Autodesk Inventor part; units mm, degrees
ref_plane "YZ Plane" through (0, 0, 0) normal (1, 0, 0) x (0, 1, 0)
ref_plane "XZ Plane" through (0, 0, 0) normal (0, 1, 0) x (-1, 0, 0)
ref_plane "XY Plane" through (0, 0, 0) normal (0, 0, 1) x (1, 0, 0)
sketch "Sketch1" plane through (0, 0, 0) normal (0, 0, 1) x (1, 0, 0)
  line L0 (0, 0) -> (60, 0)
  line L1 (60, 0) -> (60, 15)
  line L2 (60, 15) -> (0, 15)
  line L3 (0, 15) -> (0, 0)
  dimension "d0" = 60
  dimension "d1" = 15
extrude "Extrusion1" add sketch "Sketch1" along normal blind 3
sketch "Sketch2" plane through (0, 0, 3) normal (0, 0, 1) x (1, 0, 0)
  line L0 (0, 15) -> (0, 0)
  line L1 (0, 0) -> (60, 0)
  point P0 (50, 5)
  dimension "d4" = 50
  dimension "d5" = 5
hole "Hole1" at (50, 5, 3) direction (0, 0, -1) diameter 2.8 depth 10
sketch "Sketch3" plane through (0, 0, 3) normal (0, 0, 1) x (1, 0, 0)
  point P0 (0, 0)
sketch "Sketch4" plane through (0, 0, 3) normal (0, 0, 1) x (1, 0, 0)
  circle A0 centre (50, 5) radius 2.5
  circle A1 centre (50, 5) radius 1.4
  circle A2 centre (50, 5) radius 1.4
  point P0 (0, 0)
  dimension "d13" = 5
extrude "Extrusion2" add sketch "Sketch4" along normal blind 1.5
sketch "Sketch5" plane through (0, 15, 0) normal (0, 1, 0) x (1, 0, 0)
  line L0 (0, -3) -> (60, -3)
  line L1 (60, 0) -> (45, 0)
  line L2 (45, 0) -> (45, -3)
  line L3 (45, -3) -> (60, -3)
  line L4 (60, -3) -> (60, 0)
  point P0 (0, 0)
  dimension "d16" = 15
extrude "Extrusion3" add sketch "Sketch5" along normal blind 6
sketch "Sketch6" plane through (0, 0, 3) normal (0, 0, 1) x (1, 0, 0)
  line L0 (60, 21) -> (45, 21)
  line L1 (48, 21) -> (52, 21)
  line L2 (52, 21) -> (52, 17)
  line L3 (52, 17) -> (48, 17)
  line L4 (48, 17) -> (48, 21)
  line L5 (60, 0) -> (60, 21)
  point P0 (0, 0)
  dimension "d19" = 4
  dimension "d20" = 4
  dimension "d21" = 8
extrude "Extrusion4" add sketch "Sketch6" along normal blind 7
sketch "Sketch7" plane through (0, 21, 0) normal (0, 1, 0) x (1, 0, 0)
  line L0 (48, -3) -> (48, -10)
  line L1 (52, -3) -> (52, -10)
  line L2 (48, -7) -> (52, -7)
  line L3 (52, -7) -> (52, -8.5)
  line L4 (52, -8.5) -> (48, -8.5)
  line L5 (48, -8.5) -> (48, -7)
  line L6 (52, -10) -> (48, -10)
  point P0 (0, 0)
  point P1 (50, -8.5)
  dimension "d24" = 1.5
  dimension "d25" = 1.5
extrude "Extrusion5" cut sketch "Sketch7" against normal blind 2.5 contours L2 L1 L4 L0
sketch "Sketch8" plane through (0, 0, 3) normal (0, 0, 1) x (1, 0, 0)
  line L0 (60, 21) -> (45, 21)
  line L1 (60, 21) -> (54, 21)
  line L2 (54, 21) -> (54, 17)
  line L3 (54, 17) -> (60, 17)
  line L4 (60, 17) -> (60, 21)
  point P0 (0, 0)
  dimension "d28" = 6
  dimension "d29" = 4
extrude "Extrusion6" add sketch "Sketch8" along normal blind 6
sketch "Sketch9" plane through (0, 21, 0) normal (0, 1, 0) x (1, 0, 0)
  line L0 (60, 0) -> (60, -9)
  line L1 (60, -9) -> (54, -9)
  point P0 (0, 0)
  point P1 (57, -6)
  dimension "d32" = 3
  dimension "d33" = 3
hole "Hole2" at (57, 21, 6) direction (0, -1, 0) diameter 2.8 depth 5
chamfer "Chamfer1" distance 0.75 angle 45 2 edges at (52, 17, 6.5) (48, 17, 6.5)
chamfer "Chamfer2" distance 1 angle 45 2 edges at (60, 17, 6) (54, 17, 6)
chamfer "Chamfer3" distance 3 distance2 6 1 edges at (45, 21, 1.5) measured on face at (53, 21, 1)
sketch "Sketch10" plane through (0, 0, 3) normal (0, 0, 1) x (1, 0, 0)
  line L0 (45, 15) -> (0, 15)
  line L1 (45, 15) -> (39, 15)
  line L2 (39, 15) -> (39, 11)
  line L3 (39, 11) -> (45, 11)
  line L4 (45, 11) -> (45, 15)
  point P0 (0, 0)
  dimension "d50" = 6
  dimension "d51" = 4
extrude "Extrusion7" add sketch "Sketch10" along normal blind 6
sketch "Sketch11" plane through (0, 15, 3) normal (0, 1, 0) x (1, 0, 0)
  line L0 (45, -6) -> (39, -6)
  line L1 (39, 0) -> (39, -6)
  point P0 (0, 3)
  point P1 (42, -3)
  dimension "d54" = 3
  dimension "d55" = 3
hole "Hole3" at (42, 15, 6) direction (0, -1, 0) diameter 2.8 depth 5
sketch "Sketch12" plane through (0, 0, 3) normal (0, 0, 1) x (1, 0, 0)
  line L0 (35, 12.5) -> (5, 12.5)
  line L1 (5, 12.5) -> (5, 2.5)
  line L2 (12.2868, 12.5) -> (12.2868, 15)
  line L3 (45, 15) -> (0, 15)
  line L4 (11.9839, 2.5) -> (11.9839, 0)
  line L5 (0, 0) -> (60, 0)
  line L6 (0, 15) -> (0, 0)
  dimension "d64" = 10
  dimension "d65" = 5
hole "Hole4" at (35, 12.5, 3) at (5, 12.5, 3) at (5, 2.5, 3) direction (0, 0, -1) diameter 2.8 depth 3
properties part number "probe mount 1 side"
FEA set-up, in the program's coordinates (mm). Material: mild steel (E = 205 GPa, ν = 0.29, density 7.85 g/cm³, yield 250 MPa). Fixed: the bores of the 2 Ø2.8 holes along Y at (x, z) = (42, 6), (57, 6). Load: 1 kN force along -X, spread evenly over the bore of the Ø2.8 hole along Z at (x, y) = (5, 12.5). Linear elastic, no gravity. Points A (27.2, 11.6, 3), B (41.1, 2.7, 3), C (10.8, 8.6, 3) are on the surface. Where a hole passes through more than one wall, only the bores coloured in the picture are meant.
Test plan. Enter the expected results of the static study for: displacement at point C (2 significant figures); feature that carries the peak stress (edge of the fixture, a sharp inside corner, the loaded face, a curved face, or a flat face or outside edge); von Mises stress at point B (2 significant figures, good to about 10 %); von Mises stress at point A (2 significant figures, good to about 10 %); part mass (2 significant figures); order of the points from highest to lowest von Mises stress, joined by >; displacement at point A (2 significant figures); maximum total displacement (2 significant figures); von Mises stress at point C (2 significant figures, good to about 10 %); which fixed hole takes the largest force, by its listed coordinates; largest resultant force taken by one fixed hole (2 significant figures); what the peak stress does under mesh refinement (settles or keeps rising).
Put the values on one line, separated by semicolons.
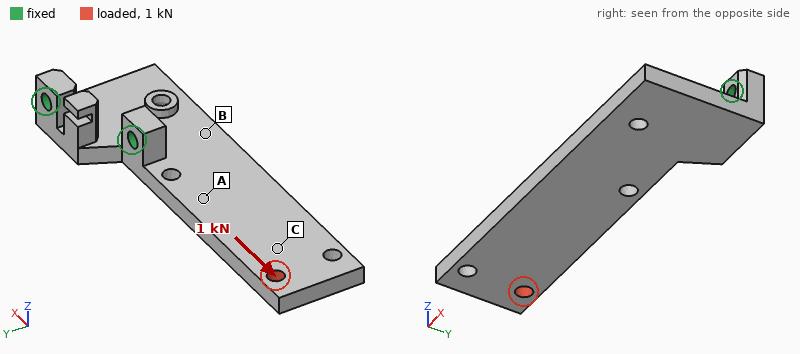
23 µm; a sharp inside corner; 13 MPa; 45 MPa; 25 g; A > C > B; 10 µm; 39 µm; 27 MPa; (42, 6); 740 N; keeps rising
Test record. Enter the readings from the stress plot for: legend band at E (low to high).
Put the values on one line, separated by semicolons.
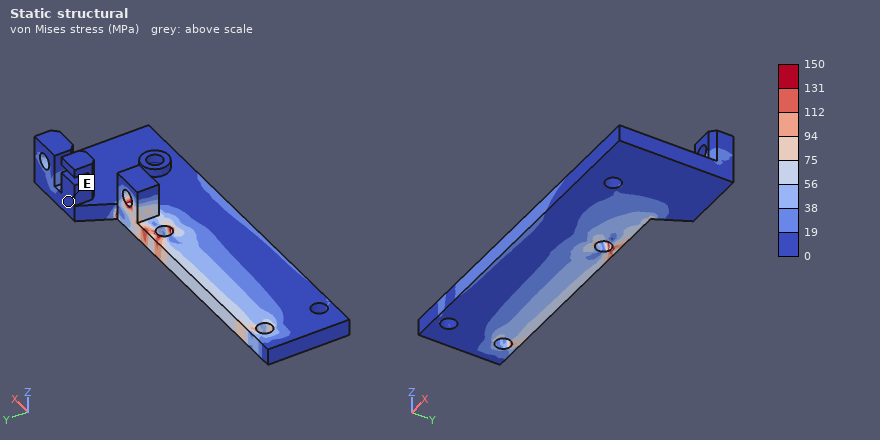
0 to 19 MPa
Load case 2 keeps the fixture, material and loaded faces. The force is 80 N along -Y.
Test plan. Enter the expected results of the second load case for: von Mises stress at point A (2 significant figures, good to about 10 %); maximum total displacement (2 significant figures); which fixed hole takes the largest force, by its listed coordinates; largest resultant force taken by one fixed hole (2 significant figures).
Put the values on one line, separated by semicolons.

8.7 MPa; 24 µm; (42, 6); 240 N
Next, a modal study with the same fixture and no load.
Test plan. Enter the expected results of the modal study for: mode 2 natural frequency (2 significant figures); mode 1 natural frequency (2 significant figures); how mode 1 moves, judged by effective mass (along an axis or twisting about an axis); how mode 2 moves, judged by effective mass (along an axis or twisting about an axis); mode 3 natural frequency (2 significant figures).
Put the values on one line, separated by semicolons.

4100 Hz; 1300 Hz; along Z; along Y; 5800 Hz
